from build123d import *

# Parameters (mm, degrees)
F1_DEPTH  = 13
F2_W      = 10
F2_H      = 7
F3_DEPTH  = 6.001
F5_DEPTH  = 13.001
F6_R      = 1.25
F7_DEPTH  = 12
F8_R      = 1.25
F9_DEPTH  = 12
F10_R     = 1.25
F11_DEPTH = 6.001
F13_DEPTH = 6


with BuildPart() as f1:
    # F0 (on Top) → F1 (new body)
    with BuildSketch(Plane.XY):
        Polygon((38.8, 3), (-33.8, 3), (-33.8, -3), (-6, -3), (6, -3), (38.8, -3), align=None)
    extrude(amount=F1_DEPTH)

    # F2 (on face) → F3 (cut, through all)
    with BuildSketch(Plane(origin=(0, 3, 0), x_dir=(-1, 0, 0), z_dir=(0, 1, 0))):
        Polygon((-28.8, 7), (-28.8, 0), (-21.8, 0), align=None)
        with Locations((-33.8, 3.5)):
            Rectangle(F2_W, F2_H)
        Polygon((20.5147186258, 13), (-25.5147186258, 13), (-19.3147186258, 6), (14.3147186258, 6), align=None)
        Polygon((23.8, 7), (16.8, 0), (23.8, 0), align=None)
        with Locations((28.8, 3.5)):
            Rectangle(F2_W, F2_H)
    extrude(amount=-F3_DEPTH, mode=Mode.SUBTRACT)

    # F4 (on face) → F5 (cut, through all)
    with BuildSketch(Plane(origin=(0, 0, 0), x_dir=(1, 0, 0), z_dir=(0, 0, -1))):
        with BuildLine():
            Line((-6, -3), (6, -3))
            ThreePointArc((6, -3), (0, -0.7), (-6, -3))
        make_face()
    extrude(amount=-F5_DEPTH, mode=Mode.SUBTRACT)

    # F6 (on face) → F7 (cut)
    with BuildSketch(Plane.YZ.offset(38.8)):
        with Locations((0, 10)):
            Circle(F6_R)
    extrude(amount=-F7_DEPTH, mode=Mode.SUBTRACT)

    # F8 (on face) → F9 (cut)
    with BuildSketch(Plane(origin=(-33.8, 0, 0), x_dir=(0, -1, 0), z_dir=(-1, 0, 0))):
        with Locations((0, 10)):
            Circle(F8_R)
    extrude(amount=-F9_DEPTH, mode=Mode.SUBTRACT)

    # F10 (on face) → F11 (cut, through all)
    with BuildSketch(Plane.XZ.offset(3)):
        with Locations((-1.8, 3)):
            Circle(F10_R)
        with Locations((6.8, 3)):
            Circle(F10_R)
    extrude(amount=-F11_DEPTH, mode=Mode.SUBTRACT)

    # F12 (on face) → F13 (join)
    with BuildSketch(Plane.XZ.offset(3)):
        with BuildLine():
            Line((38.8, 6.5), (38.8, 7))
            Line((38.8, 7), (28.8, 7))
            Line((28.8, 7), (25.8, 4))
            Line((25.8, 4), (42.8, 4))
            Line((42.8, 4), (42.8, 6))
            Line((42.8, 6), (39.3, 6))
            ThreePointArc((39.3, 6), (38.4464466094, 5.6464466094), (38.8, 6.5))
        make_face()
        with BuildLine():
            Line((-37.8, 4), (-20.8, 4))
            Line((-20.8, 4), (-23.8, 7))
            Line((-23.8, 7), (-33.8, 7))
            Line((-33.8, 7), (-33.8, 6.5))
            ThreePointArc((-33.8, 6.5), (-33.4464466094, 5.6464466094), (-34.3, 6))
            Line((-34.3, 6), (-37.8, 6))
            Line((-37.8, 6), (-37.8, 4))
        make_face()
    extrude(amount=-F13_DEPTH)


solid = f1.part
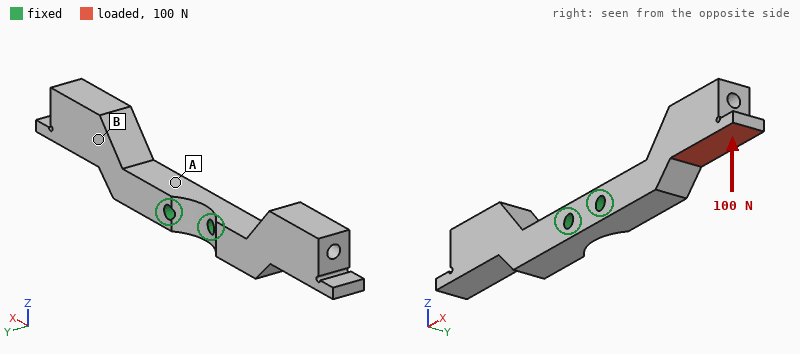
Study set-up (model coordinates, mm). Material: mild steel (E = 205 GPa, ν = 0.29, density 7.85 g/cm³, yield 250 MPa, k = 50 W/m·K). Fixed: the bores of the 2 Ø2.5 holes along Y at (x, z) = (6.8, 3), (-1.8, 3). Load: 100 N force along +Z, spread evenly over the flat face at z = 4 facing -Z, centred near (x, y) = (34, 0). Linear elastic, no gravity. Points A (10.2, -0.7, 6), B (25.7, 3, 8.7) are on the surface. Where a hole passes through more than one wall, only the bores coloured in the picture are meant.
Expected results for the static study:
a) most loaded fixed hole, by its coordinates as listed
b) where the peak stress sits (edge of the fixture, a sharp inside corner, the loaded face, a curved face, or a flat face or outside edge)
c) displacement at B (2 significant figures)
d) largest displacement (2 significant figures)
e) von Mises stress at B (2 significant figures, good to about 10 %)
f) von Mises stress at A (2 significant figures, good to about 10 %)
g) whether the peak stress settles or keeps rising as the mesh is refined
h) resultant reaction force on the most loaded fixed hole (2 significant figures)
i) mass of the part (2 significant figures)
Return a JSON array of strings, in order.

["(6.8, 3)", "edge of the fixture", "22 µm", "52 µm", "9.6 MPa", "66 MPa", "keeps rising", "180 N", "24 g"]
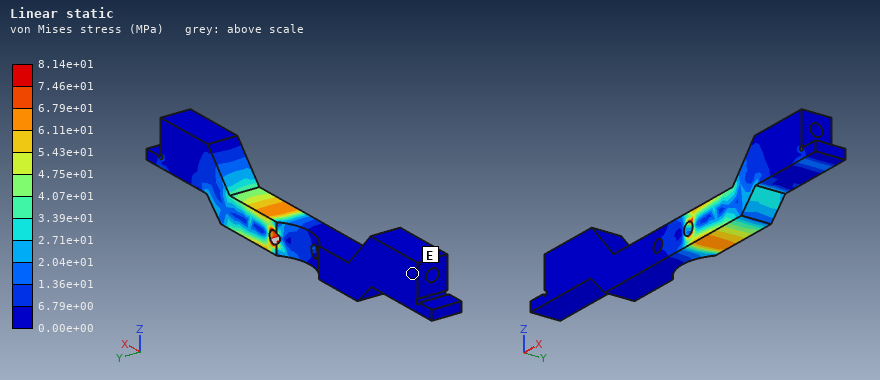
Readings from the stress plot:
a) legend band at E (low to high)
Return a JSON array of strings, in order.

["0.00e+00 to 6.79e+00 MPa"]
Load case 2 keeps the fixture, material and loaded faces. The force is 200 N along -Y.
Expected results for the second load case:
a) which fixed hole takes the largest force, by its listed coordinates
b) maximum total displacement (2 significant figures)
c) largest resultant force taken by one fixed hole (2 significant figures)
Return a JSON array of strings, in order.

["(6.8, 3)", "96 µm", "240 N"]
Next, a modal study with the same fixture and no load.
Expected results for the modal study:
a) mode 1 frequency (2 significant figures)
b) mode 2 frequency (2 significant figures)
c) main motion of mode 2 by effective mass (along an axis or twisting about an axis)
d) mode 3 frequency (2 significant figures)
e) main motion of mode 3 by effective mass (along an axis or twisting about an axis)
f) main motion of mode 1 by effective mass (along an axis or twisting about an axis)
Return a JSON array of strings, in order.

["3000 Hz", "3200 Hz", "along Z", "3500 Hz", "along Z", "along Y"]
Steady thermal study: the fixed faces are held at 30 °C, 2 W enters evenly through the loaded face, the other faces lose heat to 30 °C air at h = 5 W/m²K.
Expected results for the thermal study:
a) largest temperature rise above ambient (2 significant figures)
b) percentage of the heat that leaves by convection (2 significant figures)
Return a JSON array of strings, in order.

["31 K", "4.5 %"]
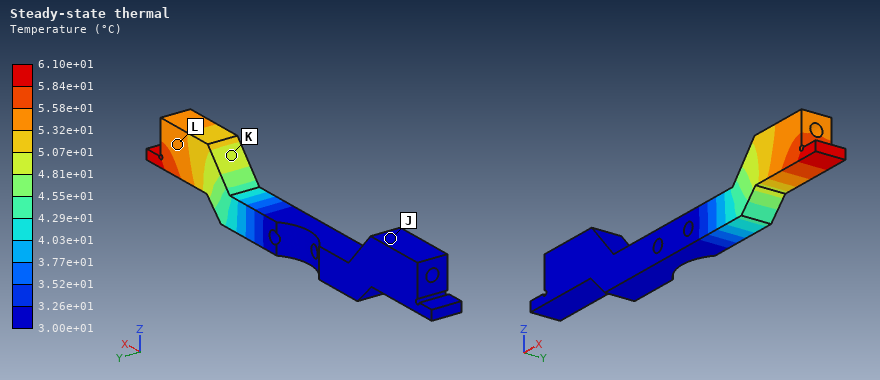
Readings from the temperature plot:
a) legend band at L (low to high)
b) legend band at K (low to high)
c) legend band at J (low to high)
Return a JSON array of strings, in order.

["5.32e+01 to 5.58e+01 °C", "4.81e+01 to 5.07e+01 °C", "3.00e+01 to 3.26e+01 °C"]
